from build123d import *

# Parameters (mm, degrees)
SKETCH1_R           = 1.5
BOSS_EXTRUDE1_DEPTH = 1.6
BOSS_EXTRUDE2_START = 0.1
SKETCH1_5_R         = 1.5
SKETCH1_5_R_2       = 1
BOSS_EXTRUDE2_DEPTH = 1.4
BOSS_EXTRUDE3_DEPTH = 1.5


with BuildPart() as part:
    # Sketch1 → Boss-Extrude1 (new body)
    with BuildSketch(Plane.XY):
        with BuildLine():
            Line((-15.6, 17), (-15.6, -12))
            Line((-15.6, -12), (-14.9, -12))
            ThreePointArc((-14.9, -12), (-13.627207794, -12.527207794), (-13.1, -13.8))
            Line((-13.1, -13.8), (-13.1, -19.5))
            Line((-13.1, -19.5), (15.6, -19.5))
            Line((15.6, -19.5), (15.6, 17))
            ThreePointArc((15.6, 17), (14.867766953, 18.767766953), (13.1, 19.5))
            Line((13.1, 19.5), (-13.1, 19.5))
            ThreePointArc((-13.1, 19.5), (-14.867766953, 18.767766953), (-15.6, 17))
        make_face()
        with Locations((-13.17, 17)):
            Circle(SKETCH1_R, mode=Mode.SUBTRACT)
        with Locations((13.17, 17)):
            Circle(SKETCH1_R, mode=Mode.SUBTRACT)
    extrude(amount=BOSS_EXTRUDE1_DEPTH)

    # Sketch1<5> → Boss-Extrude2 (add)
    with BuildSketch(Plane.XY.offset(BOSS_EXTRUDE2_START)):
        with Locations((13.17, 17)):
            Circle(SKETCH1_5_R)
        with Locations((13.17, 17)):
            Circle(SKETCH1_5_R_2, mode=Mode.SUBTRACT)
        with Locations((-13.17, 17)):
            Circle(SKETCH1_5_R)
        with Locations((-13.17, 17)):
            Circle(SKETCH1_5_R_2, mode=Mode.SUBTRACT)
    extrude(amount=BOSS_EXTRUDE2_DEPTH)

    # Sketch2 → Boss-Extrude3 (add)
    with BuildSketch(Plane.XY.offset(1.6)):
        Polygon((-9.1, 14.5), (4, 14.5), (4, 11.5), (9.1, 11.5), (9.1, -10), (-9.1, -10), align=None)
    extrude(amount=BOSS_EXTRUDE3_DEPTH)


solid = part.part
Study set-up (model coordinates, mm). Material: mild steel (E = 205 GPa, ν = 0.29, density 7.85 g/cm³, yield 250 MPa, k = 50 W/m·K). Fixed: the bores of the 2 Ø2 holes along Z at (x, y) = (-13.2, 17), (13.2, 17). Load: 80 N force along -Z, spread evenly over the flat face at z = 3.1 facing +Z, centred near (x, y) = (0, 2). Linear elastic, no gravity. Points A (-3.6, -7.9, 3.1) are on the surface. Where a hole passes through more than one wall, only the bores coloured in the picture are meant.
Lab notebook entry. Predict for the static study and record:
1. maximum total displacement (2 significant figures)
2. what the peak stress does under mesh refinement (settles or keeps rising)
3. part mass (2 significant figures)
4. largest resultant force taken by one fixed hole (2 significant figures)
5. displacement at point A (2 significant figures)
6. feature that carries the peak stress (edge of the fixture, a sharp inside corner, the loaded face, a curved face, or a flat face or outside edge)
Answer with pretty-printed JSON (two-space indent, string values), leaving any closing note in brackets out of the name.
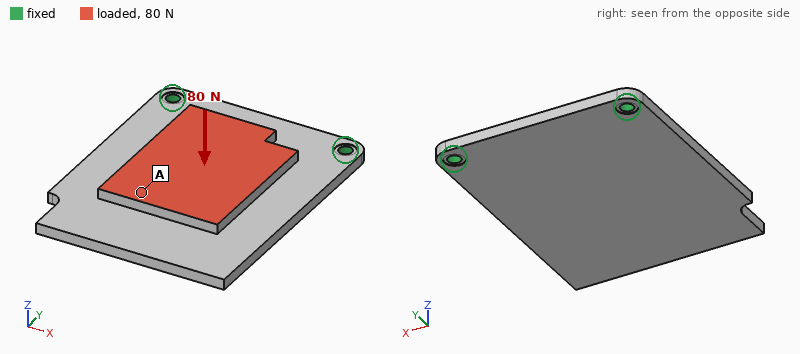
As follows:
{
  "maximum total displacement": "0.16 mm",
  "what the peak stress does under mesh refinement": "keeps rising",
  "part mass": "20 g",
  "largest resultant force taken by one fixed hole": "41 N",
  "displacement at point A": "0.10 mm",
  "feature that carries the peak stress": "edge of the fixture"
}
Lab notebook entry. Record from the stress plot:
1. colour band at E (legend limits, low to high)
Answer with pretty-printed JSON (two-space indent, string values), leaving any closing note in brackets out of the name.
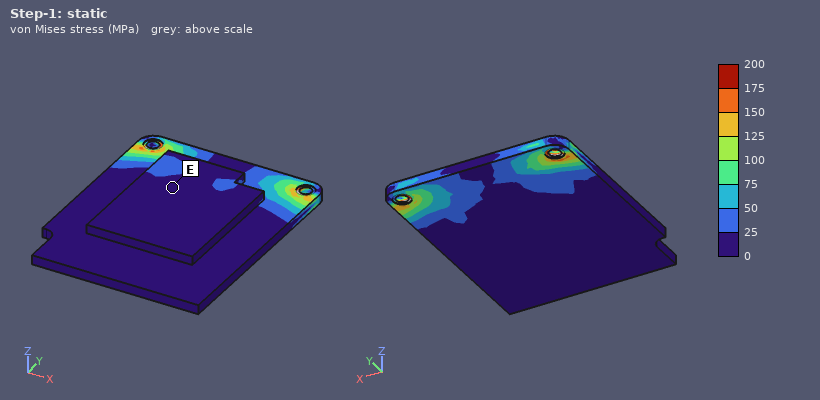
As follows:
{
  "colour band at E": "0 to 25 MPa"
}
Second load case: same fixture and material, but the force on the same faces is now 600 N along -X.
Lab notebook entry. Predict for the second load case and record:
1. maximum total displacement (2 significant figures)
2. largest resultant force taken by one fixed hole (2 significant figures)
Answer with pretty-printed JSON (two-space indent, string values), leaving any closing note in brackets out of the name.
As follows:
{
  "maximum total displacement": "17 µm",
  "largest resultant force taken by one fixed hole": "460 N"
}
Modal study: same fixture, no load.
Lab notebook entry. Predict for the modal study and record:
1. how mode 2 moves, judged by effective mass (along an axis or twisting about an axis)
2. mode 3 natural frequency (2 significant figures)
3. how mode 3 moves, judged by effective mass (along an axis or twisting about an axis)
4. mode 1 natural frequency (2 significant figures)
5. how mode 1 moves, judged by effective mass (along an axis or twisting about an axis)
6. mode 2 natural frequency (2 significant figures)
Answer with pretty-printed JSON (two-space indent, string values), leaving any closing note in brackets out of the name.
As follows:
{
  "how mode 2 moves, judged by effective mass": "twisting about Y",
  "mode 3 natural frequency": "7900 Hz",
  "how mode 3 moves, judged by effective mass": "along Z",
  "mode 1 natural frequency": "960 Hz",
  "how mode 1 moves, judged by effective mass": "along Z",
  "mode 2 natural frequency": "4600 Hz"
}
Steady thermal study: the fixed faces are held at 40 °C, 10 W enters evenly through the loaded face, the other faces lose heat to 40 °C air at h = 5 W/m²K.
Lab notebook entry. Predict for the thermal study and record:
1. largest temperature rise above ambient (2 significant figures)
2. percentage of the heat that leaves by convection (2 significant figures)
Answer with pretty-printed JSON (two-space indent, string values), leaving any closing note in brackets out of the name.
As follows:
{
  "largest temperature rise above ambient": "69 K",
  "percentage of the heat that leaves by convection": "6.1 %"
}
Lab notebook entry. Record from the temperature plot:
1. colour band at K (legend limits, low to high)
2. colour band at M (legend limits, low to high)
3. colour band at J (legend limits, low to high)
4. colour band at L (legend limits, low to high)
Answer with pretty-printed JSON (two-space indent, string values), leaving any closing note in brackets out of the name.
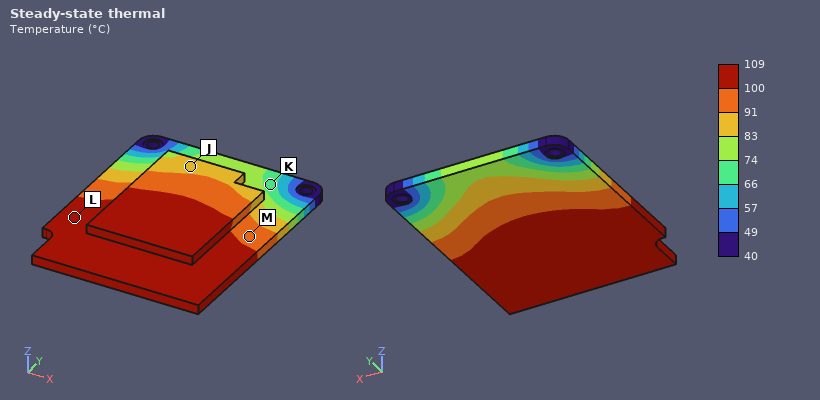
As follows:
{
  "colour band at K": "66 to 74 °C",
  "colour band at M": "91 to 100 °C",
  "colour band at J": "83 to 91 °C",
  "colour band at L": "100 to 109 °C"
}
